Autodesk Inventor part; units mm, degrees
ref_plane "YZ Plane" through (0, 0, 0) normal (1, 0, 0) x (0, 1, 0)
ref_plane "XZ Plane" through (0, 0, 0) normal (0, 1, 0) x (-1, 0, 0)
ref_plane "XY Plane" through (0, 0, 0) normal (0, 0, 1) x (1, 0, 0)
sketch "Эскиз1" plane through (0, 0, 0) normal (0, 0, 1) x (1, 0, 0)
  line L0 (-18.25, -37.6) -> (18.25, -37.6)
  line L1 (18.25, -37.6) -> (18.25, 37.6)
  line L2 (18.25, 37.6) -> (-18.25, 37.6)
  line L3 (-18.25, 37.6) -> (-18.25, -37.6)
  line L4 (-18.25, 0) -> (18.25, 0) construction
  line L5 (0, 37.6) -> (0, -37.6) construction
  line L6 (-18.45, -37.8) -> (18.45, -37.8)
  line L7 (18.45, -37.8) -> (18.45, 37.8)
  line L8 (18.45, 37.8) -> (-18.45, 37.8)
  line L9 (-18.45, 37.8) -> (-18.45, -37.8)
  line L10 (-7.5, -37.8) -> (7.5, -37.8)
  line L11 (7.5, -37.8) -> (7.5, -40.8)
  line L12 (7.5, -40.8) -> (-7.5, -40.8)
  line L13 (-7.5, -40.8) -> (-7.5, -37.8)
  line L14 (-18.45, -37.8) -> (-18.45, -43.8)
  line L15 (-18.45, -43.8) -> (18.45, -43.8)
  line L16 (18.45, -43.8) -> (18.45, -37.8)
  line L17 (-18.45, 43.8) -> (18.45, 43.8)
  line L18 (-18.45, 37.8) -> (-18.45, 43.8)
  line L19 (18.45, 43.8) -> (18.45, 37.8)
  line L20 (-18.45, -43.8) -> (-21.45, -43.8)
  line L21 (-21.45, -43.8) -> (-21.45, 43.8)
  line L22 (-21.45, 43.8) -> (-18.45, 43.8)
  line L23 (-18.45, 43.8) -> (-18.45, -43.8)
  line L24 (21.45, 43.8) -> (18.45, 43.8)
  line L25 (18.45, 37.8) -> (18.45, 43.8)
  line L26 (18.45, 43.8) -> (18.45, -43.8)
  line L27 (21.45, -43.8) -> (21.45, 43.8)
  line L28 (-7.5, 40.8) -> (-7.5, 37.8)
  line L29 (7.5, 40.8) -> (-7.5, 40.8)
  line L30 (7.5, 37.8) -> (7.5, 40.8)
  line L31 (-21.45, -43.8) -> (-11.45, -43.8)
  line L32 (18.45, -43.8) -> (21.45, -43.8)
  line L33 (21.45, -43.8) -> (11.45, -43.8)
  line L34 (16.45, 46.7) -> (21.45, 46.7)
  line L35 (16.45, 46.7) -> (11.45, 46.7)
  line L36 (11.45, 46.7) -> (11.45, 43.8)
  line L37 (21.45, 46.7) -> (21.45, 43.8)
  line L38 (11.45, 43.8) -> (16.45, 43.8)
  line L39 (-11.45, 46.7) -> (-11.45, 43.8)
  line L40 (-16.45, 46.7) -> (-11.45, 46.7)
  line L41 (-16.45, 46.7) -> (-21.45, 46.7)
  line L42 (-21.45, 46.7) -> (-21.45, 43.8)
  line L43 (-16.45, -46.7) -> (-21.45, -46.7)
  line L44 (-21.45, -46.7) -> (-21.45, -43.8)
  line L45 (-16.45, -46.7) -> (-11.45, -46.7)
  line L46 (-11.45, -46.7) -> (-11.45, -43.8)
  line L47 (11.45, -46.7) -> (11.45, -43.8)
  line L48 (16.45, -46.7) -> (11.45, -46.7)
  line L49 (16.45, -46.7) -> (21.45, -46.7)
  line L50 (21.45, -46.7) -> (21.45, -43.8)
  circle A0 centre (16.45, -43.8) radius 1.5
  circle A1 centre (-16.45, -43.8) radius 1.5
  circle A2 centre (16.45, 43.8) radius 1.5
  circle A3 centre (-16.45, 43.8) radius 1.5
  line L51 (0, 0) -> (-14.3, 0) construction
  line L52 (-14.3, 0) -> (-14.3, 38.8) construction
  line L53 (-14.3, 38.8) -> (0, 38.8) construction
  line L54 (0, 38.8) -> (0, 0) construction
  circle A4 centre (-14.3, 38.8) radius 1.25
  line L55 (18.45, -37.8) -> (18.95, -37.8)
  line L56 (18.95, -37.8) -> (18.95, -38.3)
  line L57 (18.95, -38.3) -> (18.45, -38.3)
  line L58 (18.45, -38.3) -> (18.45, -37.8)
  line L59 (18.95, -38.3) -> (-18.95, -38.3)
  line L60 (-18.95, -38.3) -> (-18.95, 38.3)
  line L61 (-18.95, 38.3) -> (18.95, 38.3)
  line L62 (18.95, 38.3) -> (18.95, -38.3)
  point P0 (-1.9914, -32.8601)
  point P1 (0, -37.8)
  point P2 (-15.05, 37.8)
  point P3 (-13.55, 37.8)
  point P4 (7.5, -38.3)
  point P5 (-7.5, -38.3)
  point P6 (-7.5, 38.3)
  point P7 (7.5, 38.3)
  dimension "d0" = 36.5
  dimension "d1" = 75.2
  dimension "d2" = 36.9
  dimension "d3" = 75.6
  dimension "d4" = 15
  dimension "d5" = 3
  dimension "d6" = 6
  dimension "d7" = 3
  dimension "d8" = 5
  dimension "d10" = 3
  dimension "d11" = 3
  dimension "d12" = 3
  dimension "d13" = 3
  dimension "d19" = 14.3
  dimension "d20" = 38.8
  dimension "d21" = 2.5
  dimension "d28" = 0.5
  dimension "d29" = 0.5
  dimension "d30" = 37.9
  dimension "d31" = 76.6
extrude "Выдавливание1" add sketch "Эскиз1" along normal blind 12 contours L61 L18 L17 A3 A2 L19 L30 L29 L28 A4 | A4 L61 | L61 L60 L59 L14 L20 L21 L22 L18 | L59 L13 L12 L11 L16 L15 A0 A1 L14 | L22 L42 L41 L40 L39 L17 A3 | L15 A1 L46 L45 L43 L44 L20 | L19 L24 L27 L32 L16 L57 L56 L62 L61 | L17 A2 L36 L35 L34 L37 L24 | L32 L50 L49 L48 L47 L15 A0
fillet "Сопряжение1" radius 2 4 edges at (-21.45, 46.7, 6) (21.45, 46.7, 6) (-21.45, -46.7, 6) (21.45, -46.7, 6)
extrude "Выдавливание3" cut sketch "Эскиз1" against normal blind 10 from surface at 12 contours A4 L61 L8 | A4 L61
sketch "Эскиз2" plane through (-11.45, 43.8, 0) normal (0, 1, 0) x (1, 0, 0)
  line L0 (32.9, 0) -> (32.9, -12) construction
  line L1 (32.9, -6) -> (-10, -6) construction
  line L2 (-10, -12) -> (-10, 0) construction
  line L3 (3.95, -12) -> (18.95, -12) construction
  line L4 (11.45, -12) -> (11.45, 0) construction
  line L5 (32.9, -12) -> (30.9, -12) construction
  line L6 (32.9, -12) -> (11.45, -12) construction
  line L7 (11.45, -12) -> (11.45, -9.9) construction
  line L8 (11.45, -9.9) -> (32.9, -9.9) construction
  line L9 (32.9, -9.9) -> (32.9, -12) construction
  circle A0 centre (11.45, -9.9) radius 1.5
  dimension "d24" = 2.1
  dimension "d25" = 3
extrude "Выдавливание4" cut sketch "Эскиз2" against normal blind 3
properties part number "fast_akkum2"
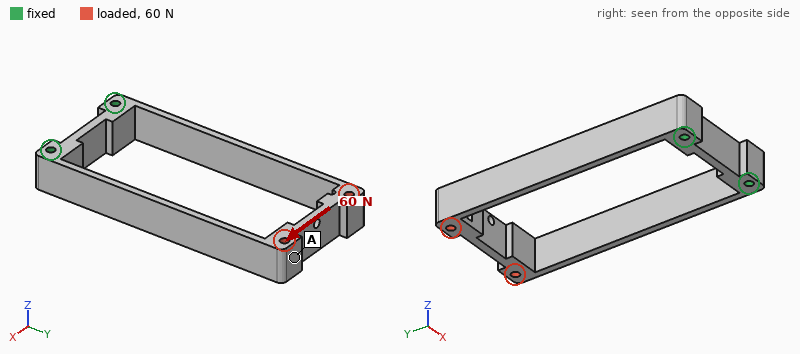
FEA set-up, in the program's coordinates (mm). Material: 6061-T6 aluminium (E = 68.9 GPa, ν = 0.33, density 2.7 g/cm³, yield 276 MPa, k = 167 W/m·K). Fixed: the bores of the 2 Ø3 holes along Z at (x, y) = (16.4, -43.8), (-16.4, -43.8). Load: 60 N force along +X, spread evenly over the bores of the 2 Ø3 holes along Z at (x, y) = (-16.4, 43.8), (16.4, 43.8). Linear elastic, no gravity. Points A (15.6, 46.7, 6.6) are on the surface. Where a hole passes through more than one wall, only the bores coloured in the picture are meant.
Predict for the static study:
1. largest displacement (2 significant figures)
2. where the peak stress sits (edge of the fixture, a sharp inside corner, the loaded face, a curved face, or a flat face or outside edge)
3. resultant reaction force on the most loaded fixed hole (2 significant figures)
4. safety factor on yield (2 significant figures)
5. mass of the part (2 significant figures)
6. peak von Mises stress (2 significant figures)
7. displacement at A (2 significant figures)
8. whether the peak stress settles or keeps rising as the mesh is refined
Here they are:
1.2 mm
a flat face or outside edge
82 N
3.0
28 g
92 MPa
1.2 mm
settles
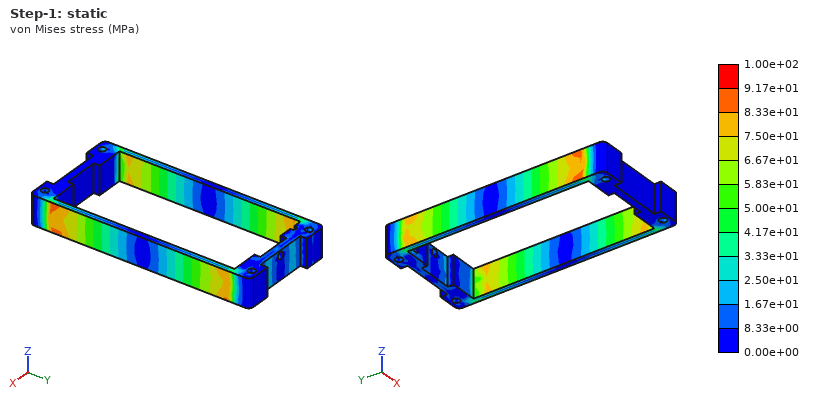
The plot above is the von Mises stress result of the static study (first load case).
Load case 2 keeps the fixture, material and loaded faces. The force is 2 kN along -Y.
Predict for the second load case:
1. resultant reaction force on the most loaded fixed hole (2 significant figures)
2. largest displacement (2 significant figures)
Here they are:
1.0 kN
0.30 mm
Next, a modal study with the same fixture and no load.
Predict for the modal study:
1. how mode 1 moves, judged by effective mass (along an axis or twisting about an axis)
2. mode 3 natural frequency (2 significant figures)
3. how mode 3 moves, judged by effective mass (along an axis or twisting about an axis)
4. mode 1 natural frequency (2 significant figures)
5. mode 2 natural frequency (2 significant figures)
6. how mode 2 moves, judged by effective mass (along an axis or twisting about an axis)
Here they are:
along X
1300 Hz
twisting about Y
320 Hz
760 Hz
along Z
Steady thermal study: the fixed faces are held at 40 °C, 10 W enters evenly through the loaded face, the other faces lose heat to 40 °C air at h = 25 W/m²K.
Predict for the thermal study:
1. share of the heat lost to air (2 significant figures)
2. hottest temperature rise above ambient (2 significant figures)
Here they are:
48 %
51 K
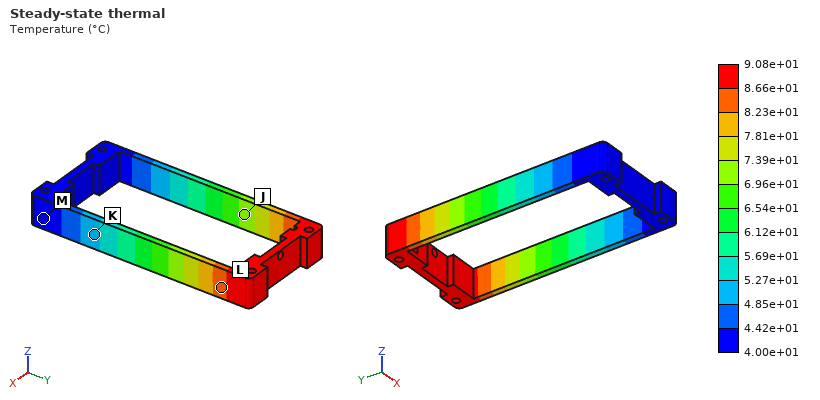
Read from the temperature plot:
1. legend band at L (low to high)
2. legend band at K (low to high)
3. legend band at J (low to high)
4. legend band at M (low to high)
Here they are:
8.23e+01 to 8.66e+01 °C
4.85e+01 to 5.27e+01 °C
6.96e+01 to 7.39e+01 °C
4.00e+01 to 4.42e+01 °C
